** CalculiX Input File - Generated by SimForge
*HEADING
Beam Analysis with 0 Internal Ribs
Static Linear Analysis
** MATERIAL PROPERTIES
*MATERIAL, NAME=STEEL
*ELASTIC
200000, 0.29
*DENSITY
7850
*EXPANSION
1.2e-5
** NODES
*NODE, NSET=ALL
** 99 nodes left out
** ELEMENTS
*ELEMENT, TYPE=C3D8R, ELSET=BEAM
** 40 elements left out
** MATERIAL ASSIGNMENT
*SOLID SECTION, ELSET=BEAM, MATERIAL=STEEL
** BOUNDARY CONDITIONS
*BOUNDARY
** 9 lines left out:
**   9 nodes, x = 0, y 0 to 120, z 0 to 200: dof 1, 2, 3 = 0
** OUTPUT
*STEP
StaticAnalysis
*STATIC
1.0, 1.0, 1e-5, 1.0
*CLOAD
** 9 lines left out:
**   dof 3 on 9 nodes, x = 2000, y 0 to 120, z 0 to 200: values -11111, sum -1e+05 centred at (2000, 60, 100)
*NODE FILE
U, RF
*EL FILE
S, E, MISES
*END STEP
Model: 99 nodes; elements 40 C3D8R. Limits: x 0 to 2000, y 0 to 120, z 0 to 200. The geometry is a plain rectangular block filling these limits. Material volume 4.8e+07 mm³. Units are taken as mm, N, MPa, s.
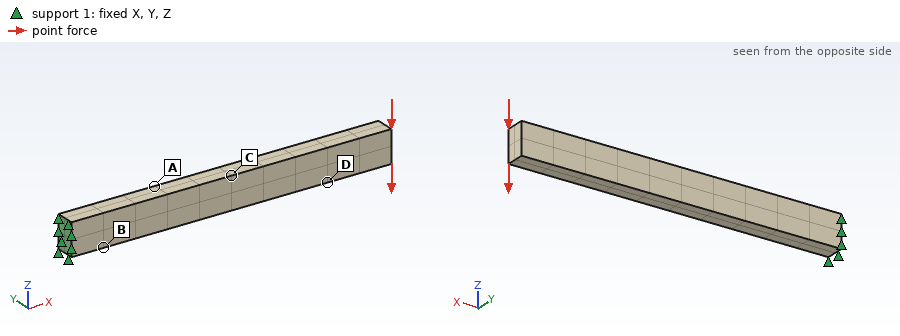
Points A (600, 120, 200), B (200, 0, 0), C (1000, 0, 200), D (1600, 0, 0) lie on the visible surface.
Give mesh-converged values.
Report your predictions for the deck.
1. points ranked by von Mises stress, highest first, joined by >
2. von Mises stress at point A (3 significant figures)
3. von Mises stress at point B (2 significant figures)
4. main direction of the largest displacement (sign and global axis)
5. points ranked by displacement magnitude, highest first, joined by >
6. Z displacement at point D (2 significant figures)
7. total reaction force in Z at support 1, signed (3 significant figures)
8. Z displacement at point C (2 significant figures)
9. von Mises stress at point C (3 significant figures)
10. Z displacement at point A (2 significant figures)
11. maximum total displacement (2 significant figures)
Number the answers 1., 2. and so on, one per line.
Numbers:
1. B > A > C > D
2. 175 MPa
3. 220 MPa
4. -Z
5. D > C > A > B
6. -12 mm
7. 100000 N
8. -5.2 mm
9. 125 MPa
10. -2.0 mm
11. 17 mm
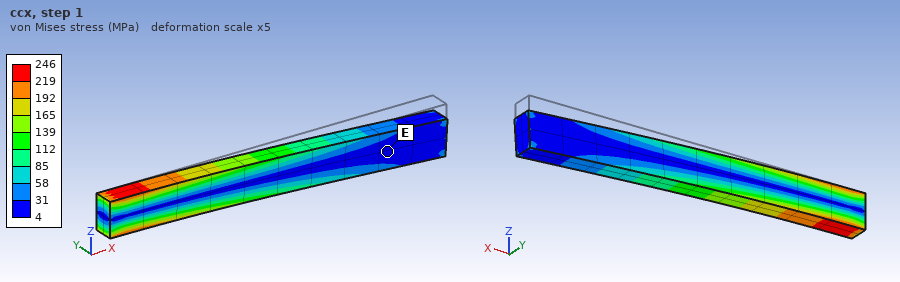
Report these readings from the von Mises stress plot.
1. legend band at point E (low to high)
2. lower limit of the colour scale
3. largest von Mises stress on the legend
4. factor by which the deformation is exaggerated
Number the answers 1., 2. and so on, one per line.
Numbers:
1. 4 to 31 MPa
2. 4 MPa
3. 246 MPa
4. 5
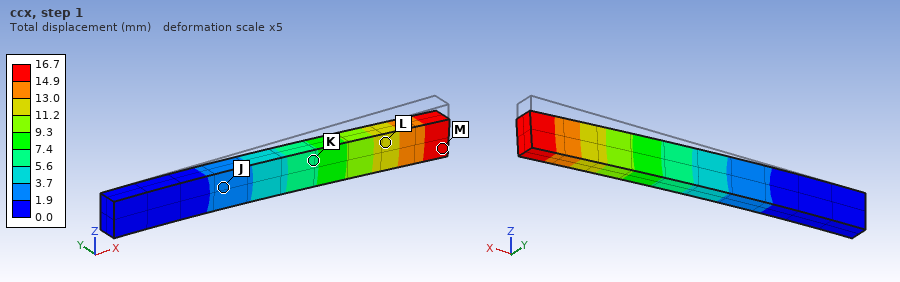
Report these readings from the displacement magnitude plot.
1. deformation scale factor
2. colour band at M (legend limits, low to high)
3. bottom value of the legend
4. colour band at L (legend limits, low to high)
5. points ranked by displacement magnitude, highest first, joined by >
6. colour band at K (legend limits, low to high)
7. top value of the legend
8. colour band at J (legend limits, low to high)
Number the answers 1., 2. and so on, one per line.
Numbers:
1. 5
2. 14.9 to 16.7 mm
3. 0.0 mm
4. 11.2 to 13.0 mm
5. M > L > K > J
6. 5.6 to 7.4 mm
7. 16.7 mm
8. 1.9 to 3.7 mm
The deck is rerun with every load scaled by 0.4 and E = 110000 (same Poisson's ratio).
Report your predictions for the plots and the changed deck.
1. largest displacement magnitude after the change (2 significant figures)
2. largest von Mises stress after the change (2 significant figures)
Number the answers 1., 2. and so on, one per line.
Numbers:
1. 12 mm
2. 98 MPa
